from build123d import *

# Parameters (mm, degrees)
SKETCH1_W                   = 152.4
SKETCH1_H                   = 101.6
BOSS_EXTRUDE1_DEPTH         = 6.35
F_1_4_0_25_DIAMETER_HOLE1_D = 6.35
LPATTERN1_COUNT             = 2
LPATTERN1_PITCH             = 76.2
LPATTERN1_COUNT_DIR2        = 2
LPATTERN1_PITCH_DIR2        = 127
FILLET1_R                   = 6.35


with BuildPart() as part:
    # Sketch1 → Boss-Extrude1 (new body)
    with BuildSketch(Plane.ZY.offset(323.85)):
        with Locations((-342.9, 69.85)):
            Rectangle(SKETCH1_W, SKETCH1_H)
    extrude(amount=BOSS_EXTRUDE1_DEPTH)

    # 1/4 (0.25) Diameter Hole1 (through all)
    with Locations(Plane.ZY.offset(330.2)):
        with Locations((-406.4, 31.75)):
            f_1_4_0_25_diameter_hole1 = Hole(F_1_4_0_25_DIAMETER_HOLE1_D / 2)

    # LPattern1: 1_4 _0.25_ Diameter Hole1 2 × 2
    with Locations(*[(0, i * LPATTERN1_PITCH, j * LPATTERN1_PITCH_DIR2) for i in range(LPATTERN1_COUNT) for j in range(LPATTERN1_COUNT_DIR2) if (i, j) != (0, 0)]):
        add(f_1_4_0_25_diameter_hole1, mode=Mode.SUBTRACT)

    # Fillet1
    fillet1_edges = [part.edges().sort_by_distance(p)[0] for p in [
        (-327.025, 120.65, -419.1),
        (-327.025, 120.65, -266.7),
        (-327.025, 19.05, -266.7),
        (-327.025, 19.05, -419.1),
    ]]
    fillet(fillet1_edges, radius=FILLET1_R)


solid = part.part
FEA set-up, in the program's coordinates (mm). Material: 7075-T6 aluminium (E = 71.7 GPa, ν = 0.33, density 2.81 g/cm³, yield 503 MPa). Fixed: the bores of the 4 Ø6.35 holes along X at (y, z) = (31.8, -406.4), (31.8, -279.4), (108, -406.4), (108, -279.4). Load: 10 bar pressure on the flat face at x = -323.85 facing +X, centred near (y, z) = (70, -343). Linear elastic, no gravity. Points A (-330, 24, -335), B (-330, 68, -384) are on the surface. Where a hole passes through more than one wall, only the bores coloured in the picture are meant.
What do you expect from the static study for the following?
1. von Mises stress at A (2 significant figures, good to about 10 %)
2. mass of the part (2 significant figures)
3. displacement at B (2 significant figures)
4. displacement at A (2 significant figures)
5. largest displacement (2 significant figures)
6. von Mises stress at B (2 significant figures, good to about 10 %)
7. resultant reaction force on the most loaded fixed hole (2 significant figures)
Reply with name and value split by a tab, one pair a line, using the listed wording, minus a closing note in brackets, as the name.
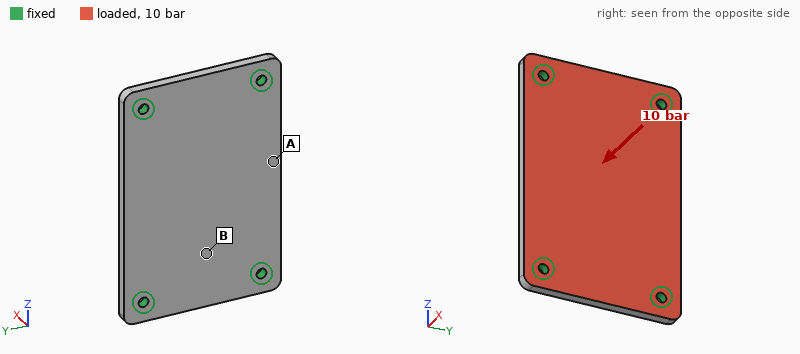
von Mises stress at A	110 MPa
mass of the part	270 g
displacement at B	0.30 mm
displacement at A	0.53 mm
largest displacement	0.59 mm
von Mises stress at B	47 MPa
resultant reaction force on the most loaded fixed hole	3.8 kN
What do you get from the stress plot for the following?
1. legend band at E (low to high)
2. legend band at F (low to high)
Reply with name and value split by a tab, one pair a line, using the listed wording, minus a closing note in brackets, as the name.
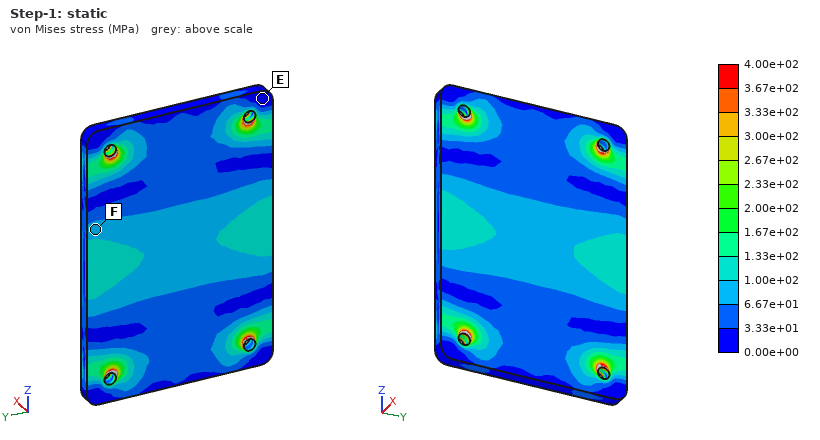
legend band at E	0.00e+00 to 3.33e+01 MPa
legend band at F	6.67e+01 to 1.00e+02 MPa
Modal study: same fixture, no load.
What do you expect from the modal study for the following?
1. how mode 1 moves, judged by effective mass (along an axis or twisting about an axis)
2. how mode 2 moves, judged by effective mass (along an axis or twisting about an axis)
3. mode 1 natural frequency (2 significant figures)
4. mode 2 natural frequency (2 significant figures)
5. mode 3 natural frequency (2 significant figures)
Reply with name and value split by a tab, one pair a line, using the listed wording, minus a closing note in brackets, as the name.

how mode 1 moves, judged by effective mass	along X
how mode 2 moves, judged by effective mass	twisting about Z
mode 1 natural frequency	1800 Hz
mode 2 natural frequency	2600 Hz
mode 3 natural frequency	4400 Hz
